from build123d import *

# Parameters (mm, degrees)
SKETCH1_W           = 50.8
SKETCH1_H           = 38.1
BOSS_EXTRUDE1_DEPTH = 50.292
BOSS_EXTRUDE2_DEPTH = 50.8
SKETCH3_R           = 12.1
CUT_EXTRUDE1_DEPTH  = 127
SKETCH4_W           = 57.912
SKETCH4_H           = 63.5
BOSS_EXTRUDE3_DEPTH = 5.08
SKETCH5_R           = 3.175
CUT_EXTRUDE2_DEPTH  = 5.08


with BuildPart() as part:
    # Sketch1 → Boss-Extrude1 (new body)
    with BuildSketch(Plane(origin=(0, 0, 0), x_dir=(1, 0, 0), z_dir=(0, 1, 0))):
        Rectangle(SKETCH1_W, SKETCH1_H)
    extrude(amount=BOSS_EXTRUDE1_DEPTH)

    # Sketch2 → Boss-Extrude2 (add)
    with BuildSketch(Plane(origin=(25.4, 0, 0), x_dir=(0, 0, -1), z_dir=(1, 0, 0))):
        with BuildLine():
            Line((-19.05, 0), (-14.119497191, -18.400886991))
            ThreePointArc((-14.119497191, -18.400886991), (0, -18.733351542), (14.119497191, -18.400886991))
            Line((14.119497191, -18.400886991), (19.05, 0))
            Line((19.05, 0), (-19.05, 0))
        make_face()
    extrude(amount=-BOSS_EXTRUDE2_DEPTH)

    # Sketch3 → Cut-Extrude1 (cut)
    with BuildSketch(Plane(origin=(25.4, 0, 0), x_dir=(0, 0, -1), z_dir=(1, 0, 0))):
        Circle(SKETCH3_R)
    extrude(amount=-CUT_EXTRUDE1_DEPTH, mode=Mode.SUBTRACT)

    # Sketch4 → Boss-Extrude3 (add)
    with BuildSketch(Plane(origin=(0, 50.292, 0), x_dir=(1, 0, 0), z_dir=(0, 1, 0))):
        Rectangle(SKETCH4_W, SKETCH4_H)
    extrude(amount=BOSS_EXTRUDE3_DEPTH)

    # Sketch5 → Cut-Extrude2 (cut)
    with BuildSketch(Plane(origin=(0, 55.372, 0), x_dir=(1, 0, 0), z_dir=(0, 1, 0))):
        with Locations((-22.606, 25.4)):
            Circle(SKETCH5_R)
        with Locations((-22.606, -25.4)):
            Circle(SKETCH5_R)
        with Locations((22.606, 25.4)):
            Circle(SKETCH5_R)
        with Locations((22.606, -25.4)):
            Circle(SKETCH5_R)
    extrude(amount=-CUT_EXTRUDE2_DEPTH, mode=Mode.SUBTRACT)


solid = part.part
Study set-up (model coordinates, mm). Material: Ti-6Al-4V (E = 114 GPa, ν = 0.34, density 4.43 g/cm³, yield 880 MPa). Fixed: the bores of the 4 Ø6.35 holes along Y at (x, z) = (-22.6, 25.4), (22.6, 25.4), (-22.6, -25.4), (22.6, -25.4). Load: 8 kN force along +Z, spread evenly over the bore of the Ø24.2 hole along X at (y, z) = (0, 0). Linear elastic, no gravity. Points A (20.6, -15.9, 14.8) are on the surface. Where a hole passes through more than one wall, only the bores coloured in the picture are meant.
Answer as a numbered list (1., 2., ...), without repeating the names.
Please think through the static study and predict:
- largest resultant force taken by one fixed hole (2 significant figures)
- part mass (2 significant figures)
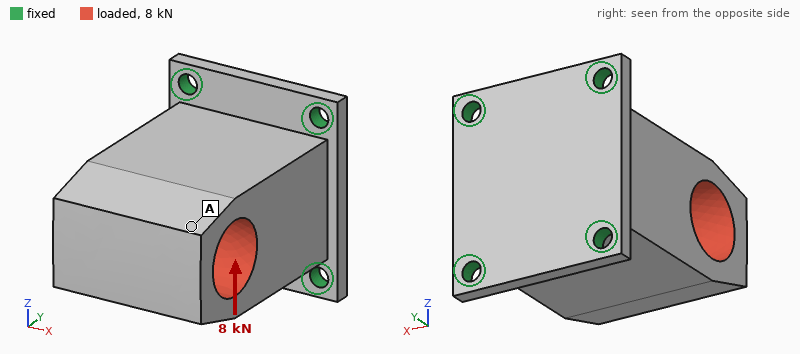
1. 5.4 kN
2. 550 g
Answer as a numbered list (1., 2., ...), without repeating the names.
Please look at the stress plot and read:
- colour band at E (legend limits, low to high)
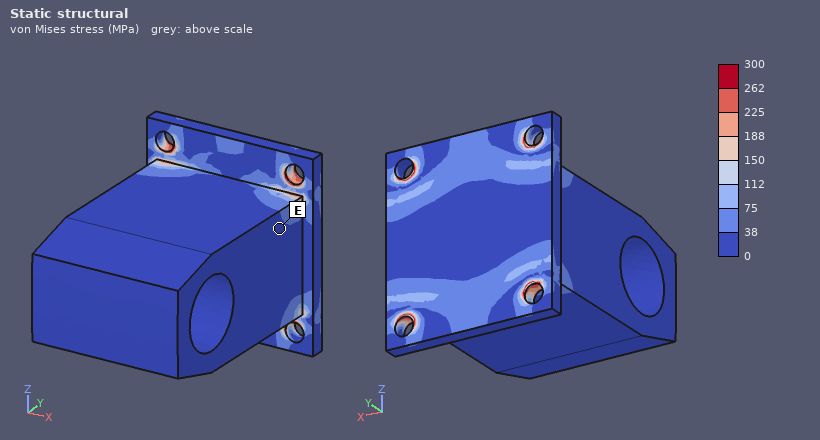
1. 0 to 38 MPa
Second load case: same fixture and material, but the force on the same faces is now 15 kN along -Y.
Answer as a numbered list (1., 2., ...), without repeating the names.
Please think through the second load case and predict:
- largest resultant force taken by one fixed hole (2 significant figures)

1. 4.1 kN
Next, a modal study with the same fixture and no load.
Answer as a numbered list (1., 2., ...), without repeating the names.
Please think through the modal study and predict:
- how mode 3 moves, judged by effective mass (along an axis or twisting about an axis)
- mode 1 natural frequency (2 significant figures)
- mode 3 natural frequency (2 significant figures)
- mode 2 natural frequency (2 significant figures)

1. along Y
2. 3200 Hz
3. 6100 Hz
4. 3300 Hz
